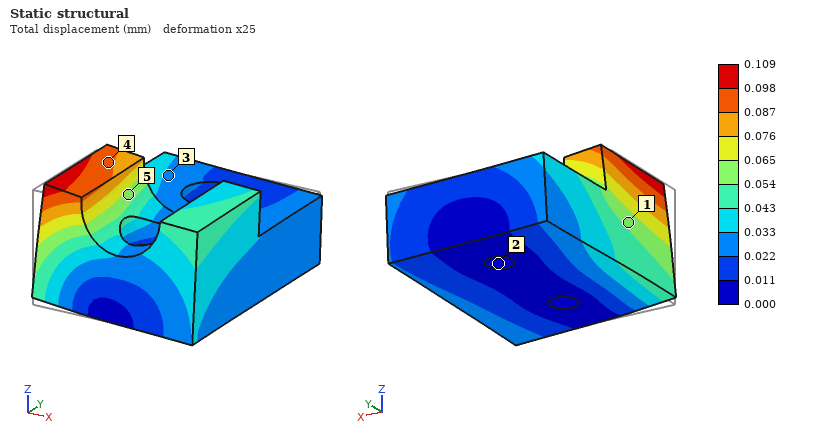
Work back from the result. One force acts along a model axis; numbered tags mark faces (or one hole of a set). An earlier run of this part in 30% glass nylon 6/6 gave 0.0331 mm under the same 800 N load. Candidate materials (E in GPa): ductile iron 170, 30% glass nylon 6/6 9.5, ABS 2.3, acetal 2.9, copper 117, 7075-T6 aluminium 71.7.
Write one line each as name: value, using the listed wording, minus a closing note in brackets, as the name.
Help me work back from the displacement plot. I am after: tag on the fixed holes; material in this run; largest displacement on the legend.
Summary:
tag on the fixed holes: 2
material in this run: acetal
largest displacement on the legend: 0.109 mm
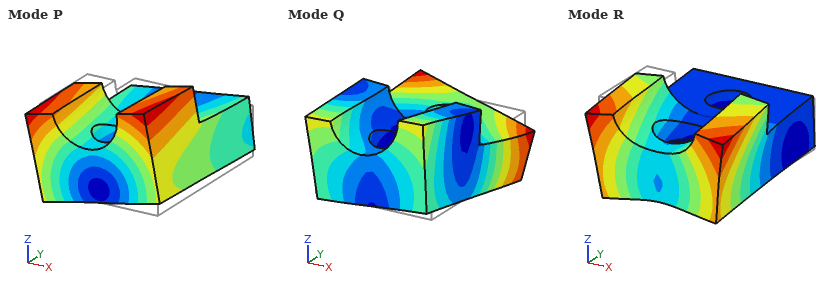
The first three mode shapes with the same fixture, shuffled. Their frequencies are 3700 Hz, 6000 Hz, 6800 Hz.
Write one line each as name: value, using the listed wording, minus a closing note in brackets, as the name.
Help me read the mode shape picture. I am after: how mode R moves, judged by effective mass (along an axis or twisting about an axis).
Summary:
how mode R moves, judged by effective mass: along Z
